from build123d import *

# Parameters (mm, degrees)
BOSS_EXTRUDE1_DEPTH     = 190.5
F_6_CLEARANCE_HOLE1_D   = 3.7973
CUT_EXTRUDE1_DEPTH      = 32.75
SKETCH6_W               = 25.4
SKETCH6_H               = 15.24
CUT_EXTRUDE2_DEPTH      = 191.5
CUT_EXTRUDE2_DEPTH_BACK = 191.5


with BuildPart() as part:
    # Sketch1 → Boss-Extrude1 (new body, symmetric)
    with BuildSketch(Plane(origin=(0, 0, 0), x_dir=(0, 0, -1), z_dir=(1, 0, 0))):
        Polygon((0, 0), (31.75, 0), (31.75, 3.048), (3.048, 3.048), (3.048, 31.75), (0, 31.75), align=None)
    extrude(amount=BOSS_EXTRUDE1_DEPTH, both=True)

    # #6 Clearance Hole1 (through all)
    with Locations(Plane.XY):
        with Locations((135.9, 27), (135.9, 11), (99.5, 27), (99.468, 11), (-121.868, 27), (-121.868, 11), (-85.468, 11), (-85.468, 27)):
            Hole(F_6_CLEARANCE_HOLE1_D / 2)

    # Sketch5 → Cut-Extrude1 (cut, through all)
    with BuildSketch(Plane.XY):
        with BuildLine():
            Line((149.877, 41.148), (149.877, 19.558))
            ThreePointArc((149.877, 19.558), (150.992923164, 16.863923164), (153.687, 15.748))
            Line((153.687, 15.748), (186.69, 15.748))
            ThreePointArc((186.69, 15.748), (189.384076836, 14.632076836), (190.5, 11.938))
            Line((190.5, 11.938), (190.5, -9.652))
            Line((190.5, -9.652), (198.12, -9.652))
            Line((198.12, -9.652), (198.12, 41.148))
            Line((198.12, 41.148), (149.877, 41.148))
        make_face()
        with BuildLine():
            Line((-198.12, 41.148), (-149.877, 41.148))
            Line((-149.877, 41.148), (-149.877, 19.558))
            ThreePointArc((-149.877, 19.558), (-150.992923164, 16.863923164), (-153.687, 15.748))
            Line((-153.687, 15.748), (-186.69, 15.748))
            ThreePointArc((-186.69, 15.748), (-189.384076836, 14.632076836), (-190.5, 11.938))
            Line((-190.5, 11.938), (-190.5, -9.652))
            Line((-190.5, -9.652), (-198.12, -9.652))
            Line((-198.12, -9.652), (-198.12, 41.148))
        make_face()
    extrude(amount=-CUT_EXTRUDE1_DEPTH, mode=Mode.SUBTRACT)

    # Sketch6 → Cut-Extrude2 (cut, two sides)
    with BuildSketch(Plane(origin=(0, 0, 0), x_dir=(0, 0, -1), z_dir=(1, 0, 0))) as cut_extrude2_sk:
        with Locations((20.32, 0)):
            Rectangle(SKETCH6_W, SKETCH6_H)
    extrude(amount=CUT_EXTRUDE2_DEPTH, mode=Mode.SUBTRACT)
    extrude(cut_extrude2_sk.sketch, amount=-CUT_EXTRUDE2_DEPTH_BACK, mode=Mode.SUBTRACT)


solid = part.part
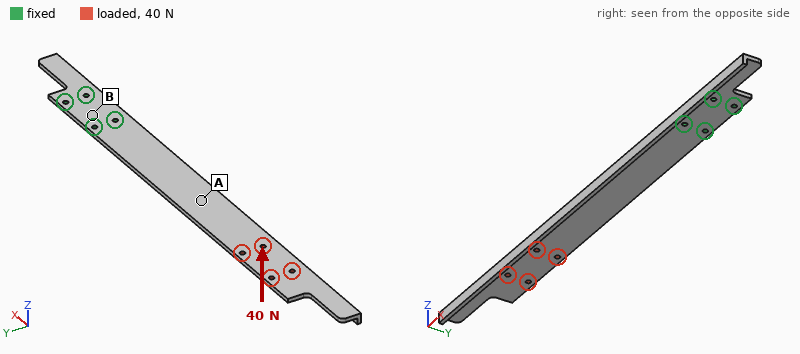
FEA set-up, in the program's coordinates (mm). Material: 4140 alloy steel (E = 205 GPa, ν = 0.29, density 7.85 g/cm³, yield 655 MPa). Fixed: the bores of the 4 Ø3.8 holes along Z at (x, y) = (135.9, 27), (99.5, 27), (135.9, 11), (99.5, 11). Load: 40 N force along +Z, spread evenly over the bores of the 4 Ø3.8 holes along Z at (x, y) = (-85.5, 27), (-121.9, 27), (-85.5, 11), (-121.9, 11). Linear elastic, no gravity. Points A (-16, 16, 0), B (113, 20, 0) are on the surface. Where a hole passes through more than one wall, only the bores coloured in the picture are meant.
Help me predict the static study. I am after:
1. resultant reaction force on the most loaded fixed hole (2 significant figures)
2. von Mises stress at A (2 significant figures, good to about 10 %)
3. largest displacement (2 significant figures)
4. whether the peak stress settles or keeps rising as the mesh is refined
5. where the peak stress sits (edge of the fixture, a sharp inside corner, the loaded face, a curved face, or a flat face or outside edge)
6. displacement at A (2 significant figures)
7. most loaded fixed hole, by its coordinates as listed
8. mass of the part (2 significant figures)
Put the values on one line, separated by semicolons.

520 N; 30 MPa; 4.0 mm; keeps rising; edge of the fixture; 1.0 mm; (99.5, 11); 300 g
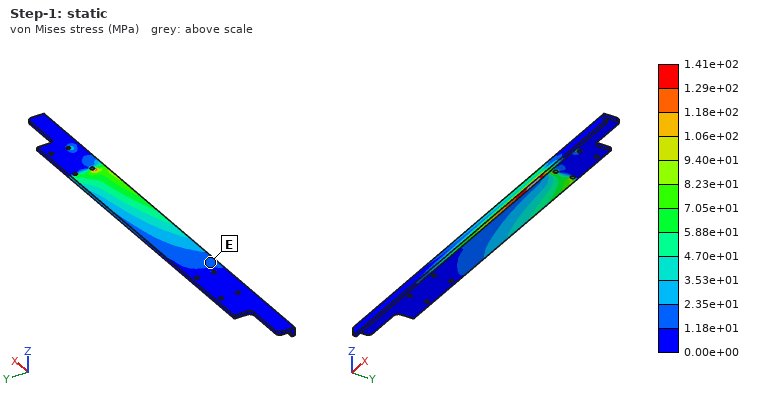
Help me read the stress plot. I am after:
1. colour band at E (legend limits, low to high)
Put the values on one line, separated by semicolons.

1.18e+01 to 2.35e+01 MPa
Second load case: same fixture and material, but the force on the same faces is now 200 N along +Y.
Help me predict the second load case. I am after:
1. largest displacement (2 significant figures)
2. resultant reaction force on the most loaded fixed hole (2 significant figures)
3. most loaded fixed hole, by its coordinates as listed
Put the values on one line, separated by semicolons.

1.3 mm; 1.8 kN; (99.5, 27)
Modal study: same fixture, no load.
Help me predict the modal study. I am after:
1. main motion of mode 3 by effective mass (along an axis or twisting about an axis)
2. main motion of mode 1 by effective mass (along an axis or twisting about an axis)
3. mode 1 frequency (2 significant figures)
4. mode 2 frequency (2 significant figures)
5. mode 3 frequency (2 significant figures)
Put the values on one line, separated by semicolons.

along Y; along Z; 54 Hz; 310 Hz; 360 Hz
